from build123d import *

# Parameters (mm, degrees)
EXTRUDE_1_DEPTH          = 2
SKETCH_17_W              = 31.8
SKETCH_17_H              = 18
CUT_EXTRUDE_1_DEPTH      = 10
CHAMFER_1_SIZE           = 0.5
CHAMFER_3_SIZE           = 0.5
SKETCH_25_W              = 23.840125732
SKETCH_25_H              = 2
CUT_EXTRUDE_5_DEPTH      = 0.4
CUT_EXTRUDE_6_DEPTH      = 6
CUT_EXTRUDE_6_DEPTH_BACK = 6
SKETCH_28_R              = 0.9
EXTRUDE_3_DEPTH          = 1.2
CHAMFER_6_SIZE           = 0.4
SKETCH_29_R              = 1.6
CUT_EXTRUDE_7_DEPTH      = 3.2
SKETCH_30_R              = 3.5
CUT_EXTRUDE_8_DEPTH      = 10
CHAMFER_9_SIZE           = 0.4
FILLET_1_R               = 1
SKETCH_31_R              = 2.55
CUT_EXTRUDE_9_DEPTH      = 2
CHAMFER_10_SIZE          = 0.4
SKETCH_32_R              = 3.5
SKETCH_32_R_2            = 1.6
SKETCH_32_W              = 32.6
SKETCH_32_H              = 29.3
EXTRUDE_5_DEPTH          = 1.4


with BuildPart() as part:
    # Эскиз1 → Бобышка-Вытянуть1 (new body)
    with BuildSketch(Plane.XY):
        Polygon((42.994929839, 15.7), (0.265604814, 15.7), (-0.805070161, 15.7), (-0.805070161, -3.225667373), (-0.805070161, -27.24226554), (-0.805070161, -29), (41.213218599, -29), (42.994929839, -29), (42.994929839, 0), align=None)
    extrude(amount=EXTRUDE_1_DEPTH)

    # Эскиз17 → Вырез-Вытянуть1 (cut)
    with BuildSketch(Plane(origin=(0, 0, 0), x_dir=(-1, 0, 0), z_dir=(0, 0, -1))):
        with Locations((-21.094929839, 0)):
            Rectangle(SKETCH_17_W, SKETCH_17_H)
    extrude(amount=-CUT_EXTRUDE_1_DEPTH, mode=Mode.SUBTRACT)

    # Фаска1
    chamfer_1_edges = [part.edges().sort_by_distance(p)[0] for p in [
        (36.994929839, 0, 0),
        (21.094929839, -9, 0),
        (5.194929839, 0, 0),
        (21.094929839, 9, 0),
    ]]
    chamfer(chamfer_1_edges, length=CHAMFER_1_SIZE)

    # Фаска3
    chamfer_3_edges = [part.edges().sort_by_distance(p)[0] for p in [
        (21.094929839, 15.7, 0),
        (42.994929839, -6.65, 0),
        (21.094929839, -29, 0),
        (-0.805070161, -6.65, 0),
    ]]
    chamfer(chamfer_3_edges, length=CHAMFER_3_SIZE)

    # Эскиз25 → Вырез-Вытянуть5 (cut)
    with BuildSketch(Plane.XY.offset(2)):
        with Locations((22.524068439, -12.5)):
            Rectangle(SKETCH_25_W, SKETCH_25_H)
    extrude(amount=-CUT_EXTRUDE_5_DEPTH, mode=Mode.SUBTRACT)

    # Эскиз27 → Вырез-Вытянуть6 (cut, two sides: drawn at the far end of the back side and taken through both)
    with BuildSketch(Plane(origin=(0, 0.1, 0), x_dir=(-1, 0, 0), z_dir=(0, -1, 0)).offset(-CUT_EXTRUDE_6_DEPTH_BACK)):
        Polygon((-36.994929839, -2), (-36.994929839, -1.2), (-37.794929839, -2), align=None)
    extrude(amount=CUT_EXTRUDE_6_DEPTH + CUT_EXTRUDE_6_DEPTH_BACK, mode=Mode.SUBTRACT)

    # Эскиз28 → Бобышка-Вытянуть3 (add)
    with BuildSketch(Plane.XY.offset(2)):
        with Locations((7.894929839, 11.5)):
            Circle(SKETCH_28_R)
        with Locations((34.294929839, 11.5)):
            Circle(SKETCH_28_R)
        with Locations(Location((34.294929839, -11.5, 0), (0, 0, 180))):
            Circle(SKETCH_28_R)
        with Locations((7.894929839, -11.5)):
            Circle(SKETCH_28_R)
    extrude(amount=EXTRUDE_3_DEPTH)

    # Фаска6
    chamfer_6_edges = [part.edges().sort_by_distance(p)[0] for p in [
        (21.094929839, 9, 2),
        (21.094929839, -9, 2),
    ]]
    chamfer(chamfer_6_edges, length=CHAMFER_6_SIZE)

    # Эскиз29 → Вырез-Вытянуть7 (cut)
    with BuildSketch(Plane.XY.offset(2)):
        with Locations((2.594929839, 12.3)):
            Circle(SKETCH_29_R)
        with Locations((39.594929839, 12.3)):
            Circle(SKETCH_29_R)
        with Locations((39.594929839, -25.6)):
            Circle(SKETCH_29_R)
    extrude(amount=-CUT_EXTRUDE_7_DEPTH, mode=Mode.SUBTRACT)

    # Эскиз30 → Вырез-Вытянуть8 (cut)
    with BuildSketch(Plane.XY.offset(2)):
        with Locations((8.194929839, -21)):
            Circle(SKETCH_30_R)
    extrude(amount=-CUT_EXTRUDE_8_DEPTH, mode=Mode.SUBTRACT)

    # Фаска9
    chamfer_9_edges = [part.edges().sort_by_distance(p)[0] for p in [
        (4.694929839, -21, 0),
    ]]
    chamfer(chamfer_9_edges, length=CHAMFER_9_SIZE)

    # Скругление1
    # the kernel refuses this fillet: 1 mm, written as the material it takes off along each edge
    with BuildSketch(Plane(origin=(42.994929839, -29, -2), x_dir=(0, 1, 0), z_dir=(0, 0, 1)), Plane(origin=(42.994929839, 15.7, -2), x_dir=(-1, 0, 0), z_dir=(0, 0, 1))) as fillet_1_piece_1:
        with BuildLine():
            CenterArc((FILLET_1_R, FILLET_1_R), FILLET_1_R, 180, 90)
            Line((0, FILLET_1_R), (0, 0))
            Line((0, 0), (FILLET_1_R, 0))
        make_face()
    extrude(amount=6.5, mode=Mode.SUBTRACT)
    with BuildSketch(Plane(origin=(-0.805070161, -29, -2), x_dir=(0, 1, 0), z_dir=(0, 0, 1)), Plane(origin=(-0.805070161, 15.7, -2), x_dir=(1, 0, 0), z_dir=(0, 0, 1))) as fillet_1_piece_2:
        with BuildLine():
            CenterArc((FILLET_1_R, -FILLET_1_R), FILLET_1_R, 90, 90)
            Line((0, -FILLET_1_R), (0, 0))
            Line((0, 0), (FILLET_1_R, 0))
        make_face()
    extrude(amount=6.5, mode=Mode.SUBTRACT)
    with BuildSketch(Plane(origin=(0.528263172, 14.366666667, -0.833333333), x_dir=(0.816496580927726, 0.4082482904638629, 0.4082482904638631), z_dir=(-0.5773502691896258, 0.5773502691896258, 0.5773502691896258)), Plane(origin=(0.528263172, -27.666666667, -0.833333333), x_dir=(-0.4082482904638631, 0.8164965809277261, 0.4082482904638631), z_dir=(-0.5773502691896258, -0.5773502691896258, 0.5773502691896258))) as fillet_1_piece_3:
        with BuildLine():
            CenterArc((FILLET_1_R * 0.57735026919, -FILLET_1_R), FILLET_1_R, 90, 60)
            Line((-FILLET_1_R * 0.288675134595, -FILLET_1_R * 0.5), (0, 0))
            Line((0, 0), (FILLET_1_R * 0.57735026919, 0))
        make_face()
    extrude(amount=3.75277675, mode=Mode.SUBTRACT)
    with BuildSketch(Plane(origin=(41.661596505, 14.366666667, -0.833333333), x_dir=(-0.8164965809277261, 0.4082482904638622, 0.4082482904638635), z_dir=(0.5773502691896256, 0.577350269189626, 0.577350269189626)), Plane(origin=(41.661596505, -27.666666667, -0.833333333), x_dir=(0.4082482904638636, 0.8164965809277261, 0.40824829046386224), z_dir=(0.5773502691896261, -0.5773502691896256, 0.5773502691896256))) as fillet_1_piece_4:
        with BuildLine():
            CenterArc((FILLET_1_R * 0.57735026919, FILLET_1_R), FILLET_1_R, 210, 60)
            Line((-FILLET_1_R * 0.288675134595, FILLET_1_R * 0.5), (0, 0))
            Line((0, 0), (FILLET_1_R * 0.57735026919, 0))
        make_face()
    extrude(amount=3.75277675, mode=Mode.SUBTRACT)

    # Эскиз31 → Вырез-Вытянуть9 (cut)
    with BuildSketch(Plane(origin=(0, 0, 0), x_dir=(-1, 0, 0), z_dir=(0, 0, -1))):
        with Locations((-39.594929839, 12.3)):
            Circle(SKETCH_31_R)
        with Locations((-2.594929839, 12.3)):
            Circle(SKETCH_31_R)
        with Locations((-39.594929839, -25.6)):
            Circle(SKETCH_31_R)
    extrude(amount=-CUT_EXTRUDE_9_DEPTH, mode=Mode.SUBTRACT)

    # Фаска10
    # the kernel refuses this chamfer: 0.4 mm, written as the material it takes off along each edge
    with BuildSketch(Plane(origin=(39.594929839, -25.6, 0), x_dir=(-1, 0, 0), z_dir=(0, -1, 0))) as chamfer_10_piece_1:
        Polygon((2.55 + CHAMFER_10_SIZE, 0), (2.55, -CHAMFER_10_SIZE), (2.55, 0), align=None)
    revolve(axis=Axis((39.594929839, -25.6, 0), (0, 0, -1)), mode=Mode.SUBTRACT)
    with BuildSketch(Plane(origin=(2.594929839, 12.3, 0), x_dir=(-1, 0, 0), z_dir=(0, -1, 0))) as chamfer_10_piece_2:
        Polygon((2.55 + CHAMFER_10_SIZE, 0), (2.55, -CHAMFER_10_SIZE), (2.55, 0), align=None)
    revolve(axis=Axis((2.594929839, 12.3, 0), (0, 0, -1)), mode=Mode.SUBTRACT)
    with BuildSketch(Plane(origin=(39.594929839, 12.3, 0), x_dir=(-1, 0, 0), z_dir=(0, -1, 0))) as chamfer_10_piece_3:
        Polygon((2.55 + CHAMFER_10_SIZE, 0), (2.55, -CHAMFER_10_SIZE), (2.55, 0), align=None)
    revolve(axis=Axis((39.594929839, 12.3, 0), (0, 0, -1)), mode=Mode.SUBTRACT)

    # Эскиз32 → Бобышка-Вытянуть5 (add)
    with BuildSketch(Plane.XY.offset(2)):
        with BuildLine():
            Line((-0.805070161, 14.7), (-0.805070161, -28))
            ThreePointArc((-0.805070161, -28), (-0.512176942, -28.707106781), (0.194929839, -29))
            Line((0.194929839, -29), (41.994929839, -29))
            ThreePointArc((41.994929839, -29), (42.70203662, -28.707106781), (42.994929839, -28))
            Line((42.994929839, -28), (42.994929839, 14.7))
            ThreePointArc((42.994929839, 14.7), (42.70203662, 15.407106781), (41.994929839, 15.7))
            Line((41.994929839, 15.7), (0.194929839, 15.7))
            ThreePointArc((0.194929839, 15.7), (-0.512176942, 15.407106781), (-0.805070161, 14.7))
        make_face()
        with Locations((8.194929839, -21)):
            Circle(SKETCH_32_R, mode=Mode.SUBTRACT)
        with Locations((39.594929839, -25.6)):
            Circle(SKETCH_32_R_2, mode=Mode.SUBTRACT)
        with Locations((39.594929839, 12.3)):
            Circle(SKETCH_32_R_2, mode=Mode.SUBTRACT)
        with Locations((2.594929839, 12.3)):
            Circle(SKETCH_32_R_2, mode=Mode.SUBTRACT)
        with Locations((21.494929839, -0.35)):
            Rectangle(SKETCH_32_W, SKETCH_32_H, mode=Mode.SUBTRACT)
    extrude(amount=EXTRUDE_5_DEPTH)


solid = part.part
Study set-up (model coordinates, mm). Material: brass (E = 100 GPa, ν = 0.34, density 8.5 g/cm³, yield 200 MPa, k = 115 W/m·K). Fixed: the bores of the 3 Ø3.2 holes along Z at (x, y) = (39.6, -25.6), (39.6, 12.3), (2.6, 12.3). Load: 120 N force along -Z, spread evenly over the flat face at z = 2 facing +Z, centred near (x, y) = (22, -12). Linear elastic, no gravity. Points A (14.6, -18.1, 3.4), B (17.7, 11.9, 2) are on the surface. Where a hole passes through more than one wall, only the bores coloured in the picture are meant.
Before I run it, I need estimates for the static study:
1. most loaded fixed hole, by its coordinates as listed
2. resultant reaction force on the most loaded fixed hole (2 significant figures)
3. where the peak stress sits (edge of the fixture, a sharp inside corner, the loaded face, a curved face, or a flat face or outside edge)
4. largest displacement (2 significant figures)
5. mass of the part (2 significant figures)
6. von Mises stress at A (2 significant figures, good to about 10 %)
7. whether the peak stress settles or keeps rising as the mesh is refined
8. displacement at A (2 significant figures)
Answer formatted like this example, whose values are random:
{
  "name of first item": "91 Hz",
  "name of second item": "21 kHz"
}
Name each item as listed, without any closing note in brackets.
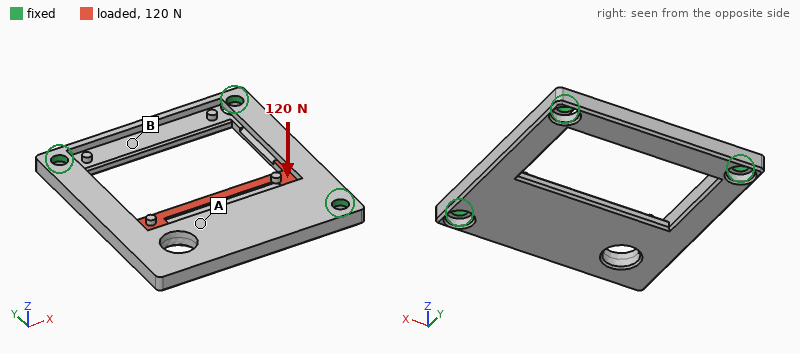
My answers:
{
  "most loaded fixed hole, by its coordinates as listed": "(39.6, -25.6)",
  "resultant reaction force on the most loaded fixed hole": "95 N",
  "where the peak stress sits": "edge of the fixture",
  "largest displacement": "70 µm",
  "mass of the part": "33 g",
  "von Mises stress at A": "21 MPa",
  "whether the peak stress settles or keeps rising as the mesh is refined": "keeps rising",
  "displacement at A": "48 µm"
}
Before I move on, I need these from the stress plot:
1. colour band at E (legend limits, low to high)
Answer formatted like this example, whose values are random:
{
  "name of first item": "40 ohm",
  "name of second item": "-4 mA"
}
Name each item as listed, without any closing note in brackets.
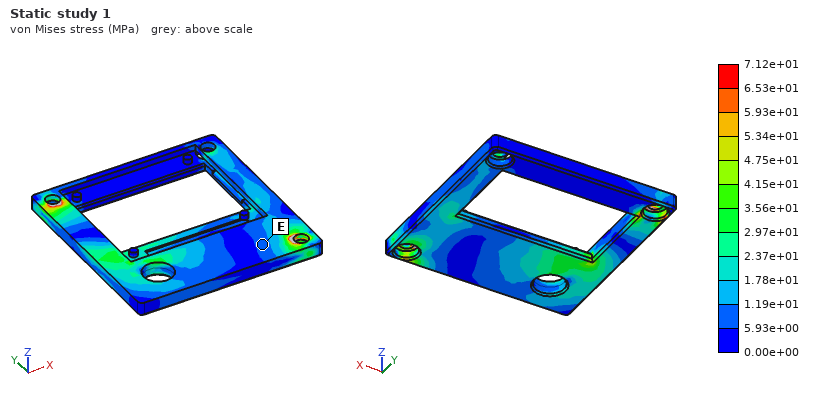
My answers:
{
  "colour band at E": "5.93e+00 to 1.19e+01 MPa"
}
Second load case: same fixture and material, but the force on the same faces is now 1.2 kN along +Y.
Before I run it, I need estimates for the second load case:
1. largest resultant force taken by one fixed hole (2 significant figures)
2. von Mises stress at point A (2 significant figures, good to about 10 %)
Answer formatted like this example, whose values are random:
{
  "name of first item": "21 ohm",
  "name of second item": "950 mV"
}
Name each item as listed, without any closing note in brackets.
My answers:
{
  "largest resultant force taken by one fixed hole": "550 N",
  "von Mises stress at point A": "14 MPa"
}
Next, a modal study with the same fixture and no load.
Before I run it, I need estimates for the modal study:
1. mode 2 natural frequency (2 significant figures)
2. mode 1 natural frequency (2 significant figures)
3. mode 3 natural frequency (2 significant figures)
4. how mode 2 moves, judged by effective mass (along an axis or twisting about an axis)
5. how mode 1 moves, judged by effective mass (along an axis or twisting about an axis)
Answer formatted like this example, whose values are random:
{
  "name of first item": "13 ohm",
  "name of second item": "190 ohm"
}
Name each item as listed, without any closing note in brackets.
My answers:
{
  "mode 2 natural frequency": "4700 Hz",
  "mode 1 natural frequency": "1400 Hz",
  "mode 3 natural frequency": "5600 Hz",
  "how mode 2 moves, judged by effective mass": "along Z",
  "how mode 1 moves, judged by effective mass": "along Z"
}
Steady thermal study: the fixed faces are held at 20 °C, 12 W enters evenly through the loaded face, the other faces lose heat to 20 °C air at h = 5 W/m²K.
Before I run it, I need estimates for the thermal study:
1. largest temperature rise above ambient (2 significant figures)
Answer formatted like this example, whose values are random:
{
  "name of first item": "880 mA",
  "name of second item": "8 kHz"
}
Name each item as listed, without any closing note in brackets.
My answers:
{
  "largest temperature rise above ambient": "34 K"
}
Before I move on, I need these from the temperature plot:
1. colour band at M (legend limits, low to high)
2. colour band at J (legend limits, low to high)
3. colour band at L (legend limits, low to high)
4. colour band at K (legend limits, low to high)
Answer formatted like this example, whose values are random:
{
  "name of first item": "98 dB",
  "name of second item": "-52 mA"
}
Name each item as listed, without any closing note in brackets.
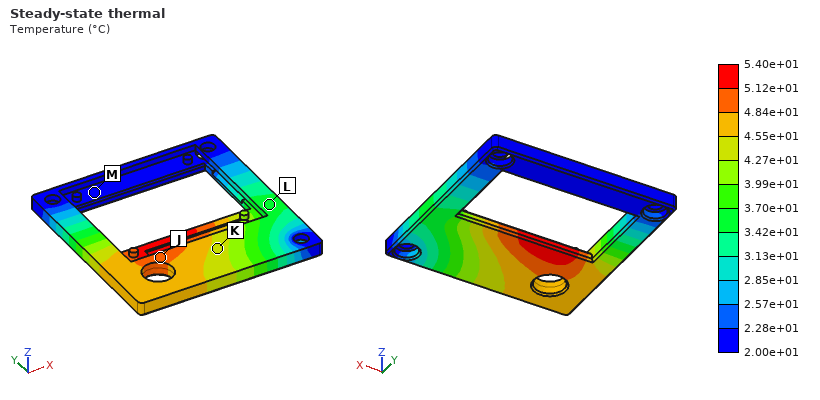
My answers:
{
  "colour band at M": "2.00e+01 to 2.28e+01 °C",
  "colour band at J": "4.84e+01 to 5.12e+01 °C",
  "colour band at L": "3.42e+01 to 3.70e+01 °C",
  "colour band at K": "4.27e+01 to 4.55e+01 °C"
}
